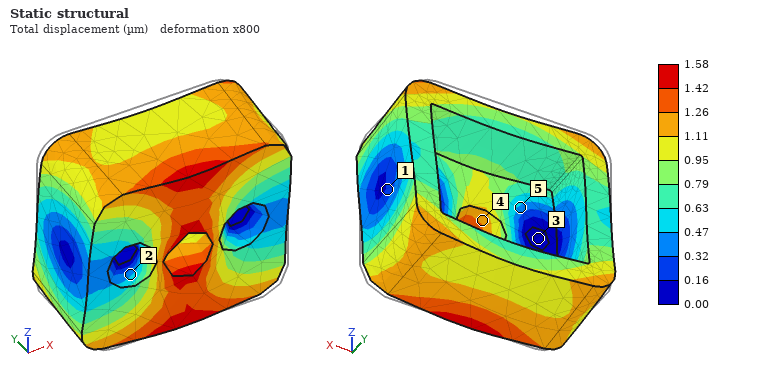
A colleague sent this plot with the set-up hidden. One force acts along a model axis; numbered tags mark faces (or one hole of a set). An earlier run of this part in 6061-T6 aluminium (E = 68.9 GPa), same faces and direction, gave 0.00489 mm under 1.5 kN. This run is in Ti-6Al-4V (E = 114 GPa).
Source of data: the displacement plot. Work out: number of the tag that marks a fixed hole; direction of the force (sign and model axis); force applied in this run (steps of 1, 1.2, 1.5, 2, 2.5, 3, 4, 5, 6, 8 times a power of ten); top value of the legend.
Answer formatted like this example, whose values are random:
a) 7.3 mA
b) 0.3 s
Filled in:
a) 3
b) -Z
c) 800 N
d) 1.58 µm
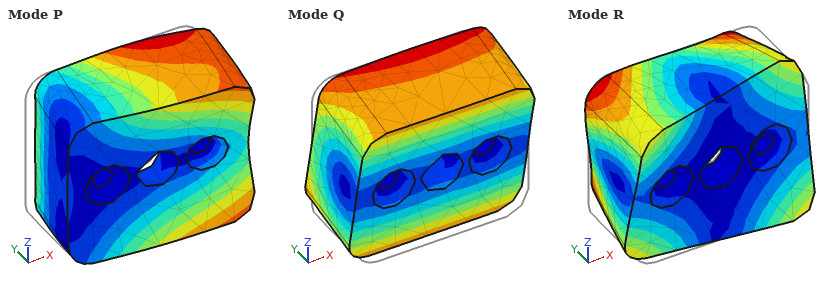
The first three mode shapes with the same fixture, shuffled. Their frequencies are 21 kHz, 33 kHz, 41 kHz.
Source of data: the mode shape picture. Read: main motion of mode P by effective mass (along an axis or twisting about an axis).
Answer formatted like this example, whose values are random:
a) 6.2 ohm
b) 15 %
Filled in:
a) along Y
